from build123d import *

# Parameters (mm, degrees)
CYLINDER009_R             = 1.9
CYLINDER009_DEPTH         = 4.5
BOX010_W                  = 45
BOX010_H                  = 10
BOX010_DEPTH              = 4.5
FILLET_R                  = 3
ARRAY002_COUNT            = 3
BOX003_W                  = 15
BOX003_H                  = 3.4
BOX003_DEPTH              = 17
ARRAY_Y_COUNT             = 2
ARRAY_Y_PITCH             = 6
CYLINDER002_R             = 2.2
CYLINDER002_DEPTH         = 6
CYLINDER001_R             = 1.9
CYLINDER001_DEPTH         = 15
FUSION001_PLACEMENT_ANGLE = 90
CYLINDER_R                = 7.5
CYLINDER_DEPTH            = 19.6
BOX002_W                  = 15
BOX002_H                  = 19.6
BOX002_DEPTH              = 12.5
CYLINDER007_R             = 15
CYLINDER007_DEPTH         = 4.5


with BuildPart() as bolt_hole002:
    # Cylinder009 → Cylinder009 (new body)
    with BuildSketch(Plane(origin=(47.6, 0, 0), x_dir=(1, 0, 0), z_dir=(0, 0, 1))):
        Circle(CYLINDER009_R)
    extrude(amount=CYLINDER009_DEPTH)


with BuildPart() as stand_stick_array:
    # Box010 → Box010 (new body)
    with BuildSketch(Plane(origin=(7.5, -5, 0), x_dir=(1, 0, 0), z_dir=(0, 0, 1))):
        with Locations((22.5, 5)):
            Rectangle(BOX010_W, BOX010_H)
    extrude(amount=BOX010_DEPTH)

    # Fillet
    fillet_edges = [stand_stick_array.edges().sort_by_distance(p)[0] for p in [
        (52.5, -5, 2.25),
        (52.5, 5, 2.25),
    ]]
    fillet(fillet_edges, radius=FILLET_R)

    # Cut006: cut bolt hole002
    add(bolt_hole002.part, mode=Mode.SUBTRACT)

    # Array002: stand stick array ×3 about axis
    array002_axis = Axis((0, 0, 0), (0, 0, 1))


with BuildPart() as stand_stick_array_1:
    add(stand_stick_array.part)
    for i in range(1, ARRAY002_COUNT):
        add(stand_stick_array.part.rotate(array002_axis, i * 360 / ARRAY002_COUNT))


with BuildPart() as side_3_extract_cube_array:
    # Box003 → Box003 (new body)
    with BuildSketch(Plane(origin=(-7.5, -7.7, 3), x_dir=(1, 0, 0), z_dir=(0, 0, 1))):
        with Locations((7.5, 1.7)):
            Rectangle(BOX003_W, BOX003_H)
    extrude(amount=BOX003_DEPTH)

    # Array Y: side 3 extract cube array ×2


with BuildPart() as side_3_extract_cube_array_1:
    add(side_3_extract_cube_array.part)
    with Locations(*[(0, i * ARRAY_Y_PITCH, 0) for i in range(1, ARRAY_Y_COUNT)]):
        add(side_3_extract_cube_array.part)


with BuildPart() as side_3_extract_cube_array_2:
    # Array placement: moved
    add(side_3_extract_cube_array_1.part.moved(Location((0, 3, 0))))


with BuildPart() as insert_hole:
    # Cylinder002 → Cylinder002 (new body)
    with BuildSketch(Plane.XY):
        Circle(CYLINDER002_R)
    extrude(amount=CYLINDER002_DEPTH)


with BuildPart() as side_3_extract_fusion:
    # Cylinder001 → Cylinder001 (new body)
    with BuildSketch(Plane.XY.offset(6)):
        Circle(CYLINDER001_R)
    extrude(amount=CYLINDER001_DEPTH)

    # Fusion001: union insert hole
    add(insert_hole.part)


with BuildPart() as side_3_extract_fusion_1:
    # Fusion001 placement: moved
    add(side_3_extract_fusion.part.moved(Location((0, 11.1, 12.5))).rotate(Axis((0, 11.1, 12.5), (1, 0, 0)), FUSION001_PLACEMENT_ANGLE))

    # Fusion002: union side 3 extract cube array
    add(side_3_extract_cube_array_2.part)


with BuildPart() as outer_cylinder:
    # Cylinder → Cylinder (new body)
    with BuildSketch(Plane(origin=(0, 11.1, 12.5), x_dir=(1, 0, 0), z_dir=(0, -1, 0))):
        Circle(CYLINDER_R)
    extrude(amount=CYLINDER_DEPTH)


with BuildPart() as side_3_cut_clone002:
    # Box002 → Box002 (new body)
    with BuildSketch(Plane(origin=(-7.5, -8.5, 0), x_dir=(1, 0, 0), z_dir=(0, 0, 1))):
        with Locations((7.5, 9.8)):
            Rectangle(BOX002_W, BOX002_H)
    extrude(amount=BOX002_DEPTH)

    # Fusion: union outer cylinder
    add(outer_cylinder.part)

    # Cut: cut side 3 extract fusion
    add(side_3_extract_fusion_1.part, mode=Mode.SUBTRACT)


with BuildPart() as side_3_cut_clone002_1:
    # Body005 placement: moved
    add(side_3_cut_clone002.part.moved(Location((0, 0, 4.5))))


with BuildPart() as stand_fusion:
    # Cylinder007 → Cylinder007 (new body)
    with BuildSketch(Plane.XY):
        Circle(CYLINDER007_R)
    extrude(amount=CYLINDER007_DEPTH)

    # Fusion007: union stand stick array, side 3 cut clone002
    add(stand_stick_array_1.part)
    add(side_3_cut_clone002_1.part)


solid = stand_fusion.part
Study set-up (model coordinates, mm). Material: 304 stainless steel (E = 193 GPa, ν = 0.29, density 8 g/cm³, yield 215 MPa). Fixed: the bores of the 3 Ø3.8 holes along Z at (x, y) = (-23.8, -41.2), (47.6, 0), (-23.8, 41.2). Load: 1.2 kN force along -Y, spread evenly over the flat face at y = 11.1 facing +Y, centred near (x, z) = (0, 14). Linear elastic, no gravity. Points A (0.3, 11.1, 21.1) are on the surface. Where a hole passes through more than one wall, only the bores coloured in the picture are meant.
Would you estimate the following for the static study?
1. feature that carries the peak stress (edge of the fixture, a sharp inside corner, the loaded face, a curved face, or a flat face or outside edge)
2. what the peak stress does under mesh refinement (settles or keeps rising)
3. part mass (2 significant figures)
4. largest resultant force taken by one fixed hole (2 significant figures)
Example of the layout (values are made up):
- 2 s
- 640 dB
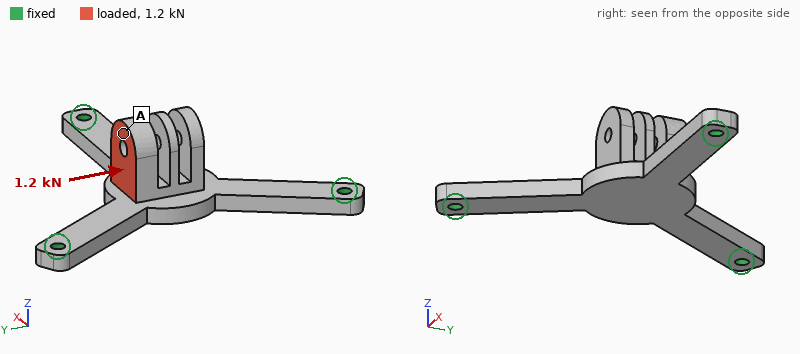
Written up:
- edge of the fixture
- keeps rising
- 94 g
- 700 N
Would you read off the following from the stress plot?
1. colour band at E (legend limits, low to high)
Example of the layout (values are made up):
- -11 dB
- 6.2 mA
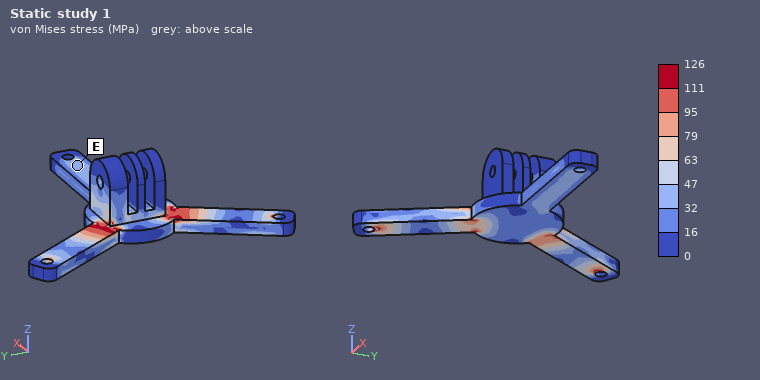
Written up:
- 32 to 47 MPa
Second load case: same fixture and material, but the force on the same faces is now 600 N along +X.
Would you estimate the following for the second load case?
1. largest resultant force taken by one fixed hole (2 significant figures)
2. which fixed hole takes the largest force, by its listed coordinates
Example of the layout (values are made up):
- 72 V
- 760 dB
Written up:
- 390 N
- (47.6, 0)
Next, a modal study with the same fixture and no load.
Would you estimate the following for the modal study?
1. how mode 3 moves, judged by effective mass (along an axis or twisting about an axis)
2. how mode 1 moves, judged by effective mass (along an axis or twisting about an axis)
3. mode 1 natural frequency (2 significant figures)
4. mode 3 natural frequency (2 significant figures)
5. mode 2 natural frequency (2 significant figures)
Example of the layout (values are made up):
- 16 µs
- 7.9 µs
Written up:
- along X
- along Z
- 1900 Hz
- 4000 Hz
- 3800 Hz
